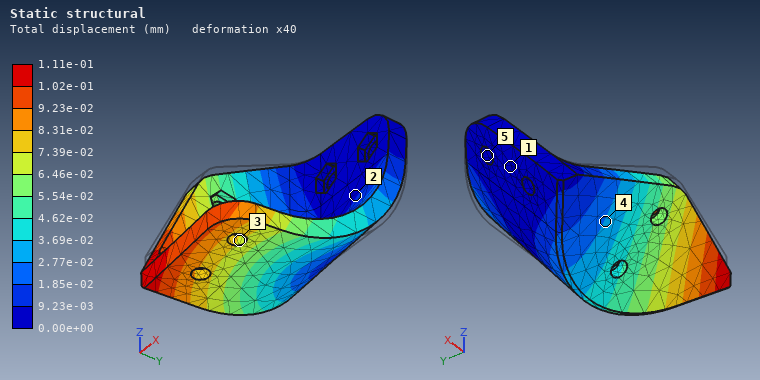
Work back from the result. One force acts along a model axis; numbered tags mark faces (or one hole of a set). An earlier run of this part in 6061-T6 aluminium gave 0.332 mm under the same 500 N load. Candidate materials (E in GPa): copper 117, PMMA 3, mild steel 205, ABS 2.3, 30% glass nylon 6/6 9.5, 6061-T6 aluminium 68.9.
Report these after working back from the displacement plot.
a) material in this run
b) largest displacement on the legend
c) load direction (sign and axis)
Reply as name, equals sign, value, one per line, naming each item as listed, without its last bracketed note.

material in this run = mild steel
largest displacement on the legend = 1.11e-01 mm
load direction = -X
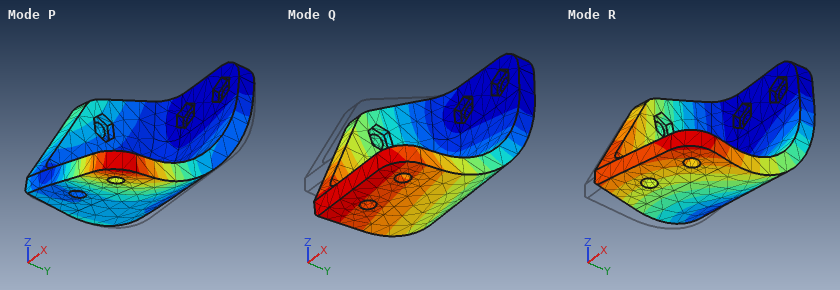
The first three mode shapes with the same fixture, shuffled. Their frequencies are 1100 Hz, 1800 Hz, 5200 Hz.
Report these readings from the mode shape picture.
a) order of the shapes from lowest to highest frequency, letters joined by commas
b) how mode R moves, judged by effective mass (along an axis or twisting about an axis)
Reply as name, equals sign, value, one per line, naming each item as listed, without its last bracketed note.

order of the shapes from lowest to highest frequency, letters joined by commas = Q, R, P
how mode R moves, judged by effective mass = along X
